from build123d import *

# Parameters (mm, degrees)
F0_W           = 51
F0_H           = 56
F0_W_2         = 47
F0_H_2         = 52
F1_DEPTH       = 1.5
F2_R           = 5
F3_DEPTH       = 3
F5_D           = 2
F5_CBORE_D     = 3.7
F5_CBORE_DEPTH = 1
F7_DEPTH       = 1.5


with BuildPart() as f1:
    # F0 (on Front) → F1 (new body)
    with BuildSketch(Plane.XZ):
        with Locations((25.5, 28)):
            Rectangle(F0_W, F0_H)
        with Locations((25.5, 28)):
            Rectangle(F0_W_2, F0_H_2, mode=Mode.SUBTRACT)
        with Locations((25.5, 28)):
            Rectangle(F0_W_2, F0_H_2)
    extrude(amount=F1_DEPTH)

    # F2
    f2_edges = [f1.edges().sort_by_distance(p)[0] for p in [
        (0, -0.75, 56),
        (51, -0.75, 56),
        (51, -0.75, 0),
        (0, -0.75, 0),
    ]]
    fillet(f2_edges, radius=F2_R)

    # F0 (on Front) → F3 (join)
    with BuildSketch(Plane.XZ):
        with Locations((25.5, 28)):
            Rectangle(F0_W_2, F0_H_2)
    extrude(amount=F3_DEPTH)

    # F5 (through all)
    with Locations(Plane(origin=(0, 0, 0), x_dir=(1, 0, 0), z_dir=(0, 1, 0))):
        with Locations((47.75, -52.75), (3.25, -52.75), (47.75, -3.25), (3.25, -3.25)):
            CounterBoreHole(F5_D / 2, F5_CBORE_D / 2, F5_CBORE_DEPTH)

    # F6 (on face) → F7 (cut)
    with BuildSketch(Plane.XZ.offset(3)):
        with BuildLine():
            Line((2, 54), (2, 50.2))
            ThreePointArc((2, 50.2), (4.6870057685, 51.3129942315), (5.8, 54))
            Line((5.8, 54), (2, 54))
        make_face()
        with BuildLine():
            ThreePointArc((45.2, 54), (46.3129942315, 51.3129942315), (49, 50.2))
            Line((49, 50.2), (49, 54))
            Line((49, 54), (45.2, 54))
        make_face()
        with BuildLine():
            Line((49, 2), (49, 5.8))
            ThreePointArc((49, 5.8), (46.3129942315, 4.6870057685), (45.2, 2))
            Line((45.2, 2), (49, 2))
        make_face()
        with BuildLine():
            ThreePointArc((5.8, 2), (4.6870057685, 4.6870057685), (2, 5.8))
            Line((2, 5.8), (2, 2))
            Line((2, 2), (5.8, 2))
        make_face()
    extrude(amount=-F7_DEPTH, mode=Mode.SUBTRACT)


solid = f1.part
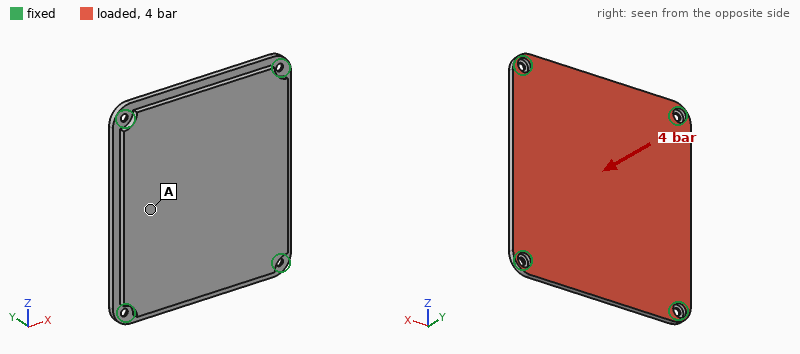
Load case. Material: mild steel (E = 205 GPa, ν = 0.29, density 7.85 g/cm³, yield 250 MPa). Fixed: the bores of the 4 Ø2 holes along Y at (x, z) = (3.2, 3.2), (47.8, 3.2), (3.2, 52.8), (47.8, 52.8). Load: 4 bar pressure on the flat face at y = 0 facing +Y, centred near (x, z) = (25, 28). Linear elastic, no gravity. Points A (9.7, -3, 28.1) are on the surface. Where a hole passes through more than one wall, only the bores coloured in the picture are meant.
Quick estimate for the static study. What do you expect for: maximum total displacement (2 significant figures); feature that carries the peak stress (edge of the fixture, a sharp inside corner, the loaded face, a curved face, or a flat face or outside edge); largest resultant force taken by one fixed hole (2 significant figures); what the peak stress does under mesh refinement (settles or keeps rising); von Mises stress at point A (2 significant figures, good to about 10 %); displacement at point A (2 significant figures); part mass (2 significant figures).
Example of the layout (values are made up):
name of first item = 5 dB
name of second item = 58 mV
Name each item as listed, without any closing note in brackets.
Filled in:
maximum total displacement = 83 µm
feature that carries the peak stress = edge of the fixture
largest resultant force taken by one fixed hole = 340 N
what the peak stress does under mesh refinement = keeps rising
von Mises stress at point A = 68 MPa
displacement at point A = 72 µm
part mass = 61 g
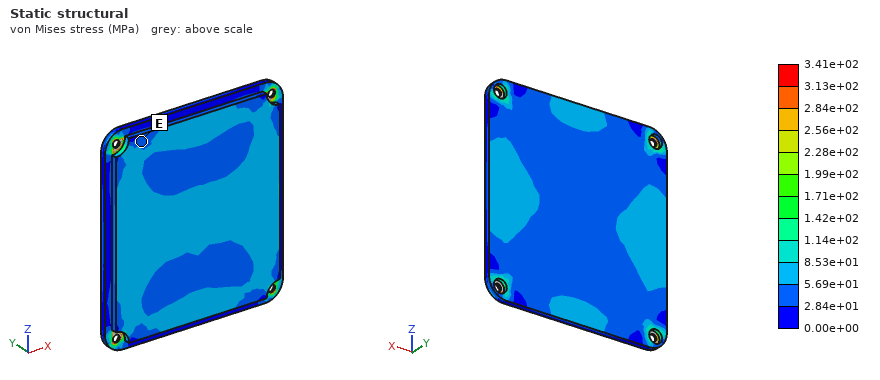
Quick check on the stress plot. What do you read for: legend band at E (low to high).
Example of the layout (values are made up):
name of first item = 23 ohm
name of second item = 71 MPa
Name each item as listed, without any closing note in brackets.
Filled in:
legend band at E = 2.84e+01 to 5.69e+01 MPa
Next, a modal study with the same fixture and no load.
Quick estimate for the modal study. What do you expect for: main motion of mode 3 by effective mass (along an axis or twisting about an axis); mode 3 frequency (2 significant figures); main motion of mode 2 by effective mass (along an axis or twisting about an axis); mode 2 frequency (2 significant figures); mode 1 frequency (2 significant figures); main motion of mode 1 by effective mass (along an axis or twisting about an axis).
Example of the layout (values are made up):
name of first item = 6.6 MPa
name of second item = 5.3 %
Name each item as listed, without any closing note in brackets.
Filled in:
main motion of mode 3 by effective mass = twisting about X
mode 3 frequency = 5500 Hz
main motion of mode 2 by effective mass = twisting about Z
mode 2 frequency = 5000 Hz
mode 1 frequency = 2700 Hz
main motion of mode 1 by effective mass = along Y
